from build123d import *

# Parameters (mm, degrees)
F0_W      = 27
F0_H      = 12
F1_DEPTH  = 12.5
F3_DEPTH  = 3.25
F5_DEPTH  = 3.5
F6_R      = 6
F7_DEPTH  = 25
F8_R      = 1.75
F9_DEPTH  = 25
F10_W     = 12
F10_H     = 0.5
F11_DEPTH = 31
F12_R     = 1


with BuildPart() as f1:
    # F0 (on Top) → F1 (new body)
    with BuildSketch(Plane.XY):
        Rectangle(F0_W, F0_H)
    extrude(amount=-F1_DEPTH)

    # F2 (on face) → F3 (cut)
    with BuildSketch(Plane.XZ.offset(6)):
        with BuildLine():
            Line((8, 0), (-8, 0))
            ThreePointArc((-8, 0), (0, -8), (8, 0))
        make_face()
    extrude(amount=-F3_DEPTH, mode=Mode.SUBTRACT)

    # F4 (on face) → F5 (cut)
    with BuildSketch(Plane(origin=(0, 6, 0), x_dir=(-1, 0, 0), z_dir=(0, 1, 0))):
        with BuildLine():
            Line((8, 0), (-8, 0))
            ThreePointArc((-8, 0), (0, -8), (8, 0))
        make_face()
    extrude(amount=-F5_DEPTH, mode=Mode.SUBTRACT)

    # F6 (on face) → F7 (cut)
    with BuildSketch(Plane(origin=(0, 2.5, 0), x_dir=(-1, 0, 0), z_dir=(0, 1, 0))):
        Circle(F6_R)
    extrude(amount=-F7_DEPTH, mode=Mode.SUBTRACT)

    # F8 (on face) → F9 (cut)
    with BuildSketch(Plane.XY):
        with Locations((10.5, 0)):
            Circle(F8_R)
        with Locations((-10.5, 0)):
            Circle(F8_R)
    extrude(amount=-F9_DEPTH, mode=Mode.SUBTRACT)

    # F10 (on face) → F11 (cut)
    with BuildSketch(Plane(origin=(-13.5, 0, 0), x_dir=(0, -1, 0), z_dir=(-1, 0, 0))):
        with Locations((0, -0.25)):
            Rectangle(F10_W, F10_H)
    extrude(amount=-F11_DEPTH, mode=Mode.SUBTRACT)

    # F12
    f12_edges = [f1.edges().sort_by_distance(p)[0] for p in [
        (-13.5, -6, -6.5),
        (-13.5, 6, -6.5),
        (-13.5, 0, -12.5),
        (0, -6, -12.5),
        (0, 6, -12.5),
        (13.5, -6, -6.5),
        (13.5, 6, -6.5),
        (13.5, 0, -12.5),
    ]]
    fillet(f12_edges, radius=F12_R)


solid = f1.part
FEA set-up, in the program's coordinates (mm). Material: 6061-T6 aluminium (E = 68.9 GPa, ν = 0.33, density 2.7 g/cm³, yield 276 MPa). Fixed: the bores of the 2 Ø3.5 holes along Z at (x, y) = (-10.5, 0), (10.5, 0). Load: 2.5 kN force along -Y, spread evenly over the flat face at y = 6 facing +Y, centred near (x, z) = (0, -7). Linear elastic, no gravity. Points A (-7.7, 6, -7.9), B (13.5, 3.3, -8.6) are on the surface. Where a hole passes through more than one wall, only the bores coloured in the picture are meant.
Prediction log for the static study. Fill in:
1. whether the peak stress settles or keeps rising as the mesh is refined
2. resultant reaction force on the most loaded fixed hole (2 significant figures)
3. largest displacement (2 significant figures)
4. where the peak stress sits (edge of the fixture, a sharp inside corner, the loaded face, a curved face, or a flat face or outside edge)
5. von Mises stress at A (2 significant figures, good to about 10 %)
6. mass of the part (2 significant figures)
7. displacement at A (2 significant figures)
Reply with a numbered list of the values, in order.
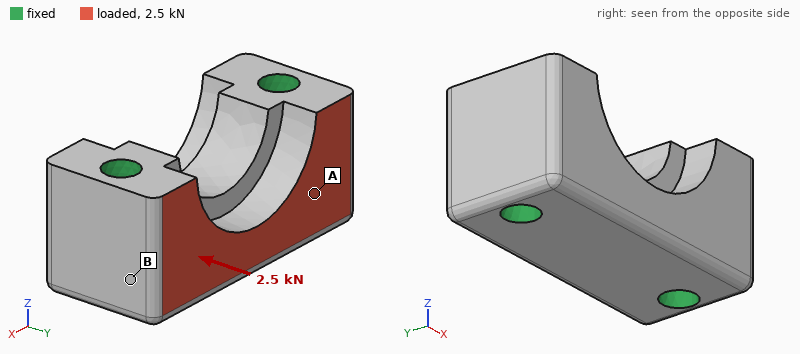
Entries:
1. keeps rising
2. 1.3 kN
3. 3.2 µm
4. edge of the fixture
5. 12 MPa
6. 7.4 g
7. 1.9 µm
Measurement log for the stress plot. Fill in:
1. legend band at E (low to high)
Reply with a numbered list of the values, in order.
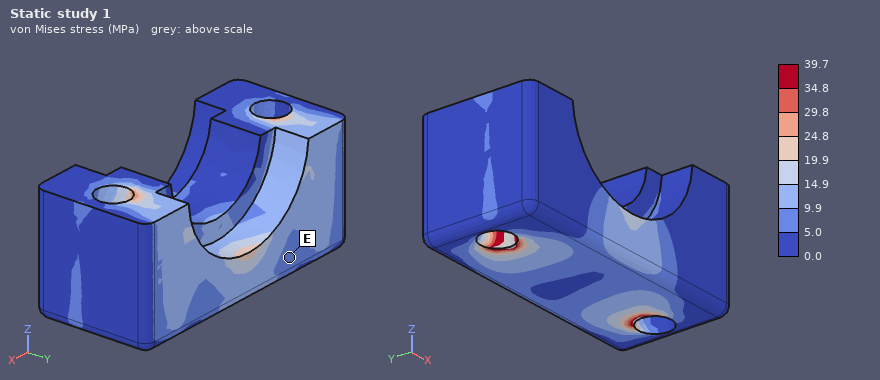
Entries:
1. 5.0 to 9.9 MPa
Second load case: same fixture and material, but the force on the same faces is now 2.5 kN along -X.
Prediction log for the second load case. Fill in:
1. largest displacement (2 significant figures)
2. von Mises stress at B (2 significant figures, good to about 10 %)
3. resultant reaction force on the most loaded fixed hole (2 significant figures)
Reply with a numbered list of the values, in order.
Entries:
1. 5.3 µm
2. 19 MPa
3. 1.3 kN
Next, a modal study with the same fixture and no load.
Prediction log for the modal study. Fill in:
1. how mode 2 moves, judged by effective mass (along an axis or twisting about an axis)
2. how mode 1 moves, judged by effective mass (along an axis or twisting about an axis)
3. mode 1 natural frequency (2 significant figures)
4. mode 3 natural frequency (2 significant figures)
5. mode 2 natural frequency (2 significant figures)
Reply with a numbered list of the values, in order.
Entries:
1. along Z
2. along Y
3. 59 kHz
4. 87 kHz
5. 71 kHz
